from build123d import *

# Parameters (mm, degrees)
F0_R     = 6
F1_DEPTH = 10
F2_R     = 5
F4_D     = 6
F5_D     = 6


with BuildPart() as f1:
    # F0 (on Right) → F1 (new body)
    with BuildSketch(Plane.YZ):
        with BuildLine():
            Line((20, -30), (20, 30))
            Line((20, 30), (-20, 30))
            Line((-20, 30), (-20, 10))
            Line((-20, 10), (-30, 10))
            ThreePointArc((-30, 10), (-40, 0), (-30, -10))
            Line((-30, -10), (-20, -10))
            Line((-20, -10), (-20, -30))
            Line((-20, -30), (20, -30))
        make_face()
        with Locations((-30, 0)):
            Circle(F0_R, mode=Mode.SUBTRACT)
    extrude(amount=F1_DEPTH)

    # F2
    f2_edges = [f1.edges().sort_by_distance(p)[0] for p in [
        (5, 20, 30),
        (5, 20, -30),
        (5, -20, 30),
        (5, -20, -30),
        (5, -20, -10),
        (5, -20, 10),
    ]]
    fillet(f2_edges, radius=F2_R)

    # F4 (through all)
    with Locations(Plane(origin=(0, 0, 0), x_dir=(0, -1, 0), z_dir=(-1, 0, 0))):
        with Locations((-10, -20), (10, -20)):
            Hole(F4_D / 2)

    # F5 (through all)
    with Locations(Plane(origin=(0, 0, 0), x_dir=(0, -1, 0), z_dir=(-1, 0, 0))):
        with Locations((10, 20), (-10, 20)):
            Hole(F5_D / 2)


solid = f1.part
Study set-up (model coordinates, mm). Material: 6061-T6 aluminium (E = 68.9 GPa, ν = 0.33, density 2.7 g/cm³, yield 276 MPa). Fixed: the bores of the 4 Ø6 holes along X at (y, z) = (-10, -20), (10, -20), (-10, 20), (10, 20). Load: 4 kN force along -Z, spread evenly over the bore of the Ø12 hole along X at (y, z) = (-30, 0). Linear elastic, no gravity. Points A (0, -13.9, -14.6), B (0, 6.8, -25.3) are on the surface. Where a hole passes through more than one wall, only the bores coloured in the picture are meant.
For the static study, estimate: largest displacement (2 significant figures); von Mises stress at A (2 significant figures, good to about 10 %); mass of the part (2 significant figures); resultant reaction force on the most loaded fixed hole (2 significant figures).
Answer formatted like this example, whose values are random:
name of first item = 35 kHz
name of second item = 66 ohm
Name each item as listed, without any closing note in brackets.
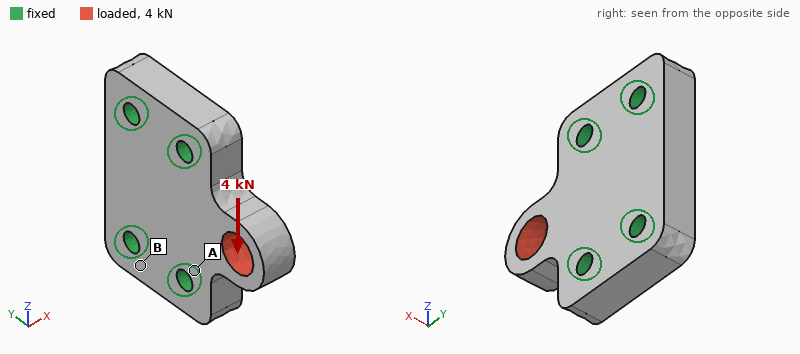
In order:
largest displacement = 63 µm
von Mises stress at A = 31 MPa
mass of the part = 68 g
resultant reaction force on the most loaded fixed hole = 2.6 kN
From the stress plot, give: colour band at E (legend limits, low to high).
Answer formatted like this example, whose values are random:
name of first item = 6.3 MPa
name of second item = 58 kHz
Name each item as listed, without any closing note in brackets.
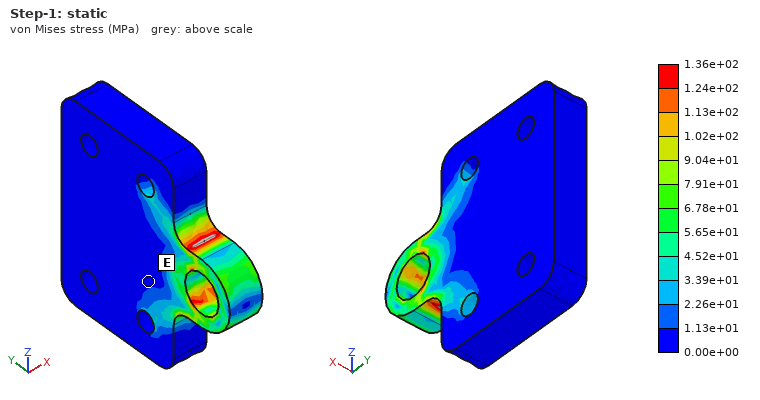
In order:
colour band at E = 0.00e+00 to 1.13e+01 MPa
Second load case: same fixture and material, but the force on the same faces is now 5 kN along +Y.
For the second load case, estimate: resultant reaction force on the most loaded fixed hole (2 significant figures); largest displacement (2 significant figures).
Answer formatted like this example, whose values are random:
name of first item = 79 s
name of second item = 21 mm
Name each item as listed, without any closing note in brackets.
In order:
resultant reaction force on the most loaded fixed hole = 1.7 kN
largest displacement = 20 µm
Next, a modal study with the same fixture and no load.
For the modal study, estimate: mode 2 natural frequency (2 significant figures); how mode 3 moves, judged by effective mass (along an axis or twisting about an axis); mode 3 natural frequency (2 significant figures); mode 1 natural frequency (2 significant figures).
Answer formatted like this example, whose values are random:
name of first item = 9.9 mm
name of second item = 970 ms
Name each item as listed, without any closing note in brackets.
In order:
mode 2 natural frequency = 19 kHz
how mode 3 moves, judged by effective mass = along X
mode 3 natural frequency = 25 kHz
mode 1 natural frequency = 10 kHz
